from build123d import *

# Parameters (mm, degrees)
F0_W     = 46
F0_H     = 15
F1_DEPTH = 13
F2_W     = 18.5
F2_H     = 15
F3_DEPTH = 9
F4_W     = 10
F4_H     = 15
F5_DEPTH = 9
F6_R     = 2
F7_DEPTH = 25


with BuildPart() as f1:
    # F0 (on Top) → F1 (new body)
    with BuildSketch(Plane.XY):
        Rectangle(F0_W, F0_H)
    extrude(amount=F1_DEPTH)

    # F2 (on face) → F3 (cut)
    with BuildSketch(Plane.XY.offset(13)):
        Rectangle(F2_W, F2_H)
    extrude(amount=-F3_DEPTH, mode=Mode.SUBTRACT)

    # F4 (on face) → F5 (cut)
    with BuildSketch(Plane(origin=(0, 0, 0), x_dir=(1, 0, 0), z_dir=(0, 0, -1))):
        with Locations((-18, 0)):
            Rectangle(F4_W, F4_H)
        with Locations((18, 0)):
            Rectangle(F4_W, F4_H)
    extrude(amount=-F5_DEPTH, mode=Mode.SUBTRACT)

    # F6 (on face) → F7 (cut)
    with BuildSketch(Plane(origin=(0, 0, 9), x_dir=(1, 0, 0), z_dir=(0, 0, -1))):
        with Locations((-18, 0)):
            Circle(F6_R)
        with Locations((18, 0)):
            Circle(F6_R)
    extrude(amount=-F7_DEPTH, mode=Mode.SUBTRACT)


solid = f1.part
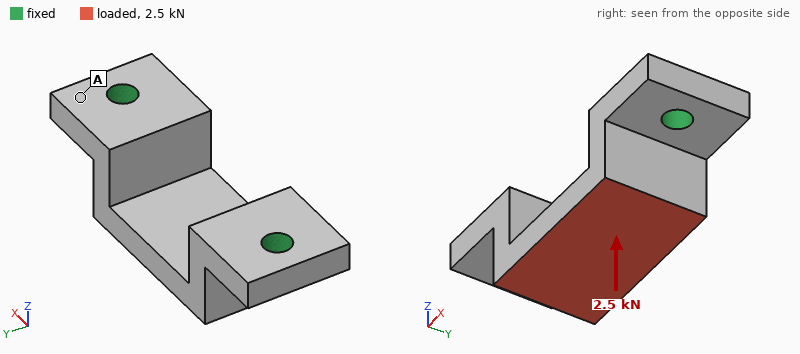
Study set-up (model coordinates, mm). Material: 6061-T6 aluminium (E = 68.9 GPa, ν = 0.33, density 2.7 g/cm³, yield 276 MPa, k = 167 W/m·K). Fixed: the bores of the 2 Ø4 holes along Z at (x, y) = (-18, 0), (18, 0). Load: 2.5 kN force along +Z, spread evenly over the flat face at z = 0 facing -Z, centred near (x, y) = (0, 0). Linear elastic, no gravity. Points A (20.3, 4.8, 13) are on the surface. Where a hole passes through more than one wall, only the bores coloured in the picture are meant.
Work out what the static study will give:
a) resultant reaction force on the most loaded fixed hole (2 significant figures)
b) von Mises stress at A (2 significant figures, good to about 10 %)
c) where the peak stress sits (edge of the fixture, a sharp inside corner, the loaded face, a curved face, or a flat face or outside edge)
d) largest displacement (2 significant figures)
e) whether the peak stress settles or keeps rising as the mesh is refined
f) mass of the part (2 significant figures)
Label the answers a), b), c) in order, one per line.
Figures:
a) 1.5 kN
b) 23 MPa
c) edge of the fixture
d) 32 µm
e) keeps rising
f) 9.9 g
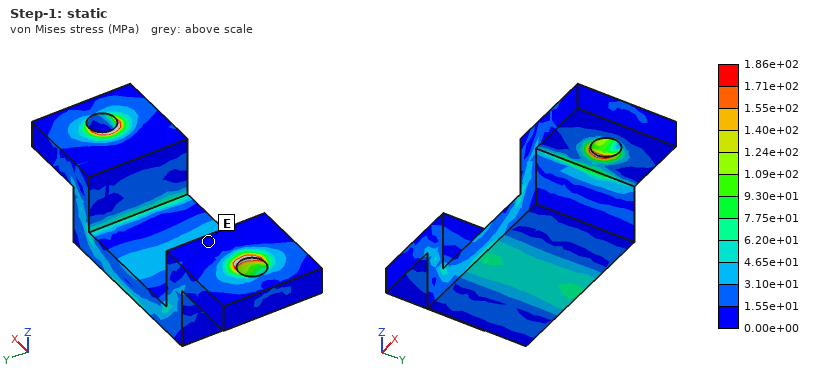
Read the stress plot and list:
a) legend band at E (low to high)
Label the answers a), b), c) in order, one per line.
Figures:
a) 0.00e+00 to 1.55e+01 MPa
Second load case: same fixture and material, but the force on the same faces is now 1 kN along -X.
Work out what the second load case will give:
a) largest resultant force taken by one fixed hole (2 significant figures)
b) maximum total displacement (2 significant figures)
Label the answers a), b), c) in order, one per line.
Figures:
a) 580 N
b) 18 µm
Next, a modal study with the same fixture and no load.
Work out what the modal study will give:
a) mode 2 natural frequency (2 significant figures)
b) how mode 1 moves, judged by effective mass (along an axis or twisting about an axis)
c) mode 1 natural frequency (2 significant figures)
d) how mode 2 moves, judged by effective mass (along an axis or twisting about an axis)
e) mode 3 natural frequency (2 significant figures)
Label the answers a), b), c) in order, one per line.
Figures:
a) 17 kHz
b) along Y
c) 11 kHz
d) along X
e) 20 kHz
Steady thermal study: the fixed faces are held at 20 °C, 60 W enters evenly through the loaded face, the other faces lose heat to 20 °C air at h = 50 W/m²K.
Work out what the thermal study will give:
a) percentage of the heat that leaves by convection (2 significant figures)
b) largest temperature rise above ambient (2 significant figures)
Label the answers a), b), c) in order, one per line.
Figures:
a) 4.0 %
b) 53 K
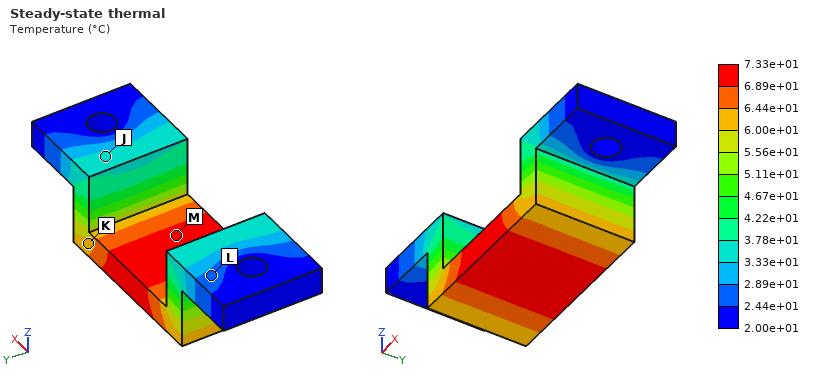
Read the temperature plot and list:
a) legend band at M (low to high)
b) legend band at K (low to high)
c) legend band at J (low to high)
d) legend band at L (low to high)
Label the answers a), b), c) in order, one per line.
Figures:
a) 6.89e+01 to 7.33e+01 °C
b) 6.00e+01 to 6.44e+01 °C
c) 3.33e+01 to 3.78e+01 °C
d) 2.44e+01 to 2.89e+01 °C
